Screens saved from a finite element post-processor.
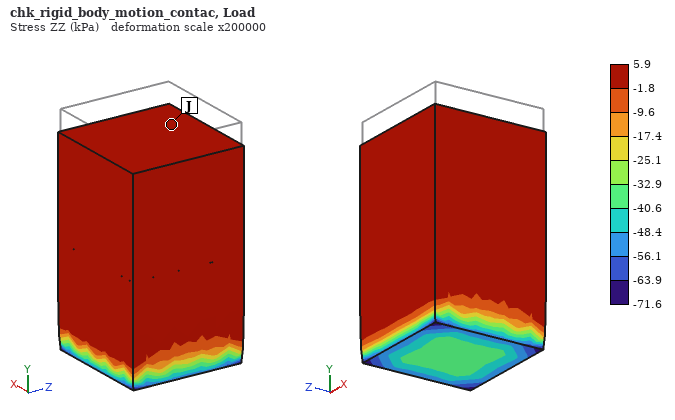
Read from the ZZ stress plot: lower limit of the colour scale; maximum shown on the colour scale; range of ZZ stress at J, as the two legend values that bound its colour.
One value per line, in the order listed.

-71.6 kPa
5.9 kPa
-1.8 to 5.9 kPa
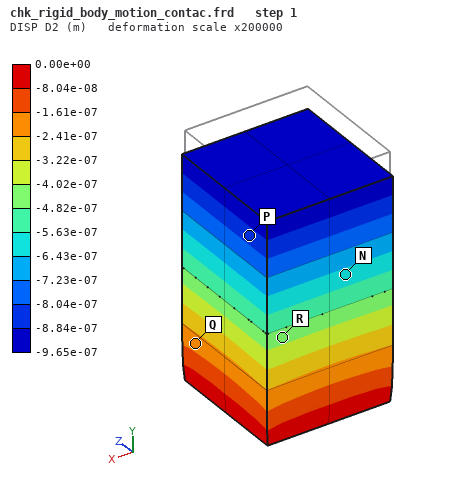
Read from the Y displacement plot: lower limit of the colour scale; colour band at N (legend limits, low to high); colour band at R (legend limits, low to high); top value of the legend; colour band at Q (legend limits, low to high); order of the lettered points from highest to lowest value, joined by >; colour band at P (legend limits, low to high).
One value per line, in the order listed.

-9.65e-07 m
-6.43e-07 to -5.63e-07 m
-4.82e-07 to -4.02e-07 m
0.00e+00 m
-2.41e-07 to -1.61e-07 m
Q > R > N > P
-8.84e-07 to -8.04e-07 m
